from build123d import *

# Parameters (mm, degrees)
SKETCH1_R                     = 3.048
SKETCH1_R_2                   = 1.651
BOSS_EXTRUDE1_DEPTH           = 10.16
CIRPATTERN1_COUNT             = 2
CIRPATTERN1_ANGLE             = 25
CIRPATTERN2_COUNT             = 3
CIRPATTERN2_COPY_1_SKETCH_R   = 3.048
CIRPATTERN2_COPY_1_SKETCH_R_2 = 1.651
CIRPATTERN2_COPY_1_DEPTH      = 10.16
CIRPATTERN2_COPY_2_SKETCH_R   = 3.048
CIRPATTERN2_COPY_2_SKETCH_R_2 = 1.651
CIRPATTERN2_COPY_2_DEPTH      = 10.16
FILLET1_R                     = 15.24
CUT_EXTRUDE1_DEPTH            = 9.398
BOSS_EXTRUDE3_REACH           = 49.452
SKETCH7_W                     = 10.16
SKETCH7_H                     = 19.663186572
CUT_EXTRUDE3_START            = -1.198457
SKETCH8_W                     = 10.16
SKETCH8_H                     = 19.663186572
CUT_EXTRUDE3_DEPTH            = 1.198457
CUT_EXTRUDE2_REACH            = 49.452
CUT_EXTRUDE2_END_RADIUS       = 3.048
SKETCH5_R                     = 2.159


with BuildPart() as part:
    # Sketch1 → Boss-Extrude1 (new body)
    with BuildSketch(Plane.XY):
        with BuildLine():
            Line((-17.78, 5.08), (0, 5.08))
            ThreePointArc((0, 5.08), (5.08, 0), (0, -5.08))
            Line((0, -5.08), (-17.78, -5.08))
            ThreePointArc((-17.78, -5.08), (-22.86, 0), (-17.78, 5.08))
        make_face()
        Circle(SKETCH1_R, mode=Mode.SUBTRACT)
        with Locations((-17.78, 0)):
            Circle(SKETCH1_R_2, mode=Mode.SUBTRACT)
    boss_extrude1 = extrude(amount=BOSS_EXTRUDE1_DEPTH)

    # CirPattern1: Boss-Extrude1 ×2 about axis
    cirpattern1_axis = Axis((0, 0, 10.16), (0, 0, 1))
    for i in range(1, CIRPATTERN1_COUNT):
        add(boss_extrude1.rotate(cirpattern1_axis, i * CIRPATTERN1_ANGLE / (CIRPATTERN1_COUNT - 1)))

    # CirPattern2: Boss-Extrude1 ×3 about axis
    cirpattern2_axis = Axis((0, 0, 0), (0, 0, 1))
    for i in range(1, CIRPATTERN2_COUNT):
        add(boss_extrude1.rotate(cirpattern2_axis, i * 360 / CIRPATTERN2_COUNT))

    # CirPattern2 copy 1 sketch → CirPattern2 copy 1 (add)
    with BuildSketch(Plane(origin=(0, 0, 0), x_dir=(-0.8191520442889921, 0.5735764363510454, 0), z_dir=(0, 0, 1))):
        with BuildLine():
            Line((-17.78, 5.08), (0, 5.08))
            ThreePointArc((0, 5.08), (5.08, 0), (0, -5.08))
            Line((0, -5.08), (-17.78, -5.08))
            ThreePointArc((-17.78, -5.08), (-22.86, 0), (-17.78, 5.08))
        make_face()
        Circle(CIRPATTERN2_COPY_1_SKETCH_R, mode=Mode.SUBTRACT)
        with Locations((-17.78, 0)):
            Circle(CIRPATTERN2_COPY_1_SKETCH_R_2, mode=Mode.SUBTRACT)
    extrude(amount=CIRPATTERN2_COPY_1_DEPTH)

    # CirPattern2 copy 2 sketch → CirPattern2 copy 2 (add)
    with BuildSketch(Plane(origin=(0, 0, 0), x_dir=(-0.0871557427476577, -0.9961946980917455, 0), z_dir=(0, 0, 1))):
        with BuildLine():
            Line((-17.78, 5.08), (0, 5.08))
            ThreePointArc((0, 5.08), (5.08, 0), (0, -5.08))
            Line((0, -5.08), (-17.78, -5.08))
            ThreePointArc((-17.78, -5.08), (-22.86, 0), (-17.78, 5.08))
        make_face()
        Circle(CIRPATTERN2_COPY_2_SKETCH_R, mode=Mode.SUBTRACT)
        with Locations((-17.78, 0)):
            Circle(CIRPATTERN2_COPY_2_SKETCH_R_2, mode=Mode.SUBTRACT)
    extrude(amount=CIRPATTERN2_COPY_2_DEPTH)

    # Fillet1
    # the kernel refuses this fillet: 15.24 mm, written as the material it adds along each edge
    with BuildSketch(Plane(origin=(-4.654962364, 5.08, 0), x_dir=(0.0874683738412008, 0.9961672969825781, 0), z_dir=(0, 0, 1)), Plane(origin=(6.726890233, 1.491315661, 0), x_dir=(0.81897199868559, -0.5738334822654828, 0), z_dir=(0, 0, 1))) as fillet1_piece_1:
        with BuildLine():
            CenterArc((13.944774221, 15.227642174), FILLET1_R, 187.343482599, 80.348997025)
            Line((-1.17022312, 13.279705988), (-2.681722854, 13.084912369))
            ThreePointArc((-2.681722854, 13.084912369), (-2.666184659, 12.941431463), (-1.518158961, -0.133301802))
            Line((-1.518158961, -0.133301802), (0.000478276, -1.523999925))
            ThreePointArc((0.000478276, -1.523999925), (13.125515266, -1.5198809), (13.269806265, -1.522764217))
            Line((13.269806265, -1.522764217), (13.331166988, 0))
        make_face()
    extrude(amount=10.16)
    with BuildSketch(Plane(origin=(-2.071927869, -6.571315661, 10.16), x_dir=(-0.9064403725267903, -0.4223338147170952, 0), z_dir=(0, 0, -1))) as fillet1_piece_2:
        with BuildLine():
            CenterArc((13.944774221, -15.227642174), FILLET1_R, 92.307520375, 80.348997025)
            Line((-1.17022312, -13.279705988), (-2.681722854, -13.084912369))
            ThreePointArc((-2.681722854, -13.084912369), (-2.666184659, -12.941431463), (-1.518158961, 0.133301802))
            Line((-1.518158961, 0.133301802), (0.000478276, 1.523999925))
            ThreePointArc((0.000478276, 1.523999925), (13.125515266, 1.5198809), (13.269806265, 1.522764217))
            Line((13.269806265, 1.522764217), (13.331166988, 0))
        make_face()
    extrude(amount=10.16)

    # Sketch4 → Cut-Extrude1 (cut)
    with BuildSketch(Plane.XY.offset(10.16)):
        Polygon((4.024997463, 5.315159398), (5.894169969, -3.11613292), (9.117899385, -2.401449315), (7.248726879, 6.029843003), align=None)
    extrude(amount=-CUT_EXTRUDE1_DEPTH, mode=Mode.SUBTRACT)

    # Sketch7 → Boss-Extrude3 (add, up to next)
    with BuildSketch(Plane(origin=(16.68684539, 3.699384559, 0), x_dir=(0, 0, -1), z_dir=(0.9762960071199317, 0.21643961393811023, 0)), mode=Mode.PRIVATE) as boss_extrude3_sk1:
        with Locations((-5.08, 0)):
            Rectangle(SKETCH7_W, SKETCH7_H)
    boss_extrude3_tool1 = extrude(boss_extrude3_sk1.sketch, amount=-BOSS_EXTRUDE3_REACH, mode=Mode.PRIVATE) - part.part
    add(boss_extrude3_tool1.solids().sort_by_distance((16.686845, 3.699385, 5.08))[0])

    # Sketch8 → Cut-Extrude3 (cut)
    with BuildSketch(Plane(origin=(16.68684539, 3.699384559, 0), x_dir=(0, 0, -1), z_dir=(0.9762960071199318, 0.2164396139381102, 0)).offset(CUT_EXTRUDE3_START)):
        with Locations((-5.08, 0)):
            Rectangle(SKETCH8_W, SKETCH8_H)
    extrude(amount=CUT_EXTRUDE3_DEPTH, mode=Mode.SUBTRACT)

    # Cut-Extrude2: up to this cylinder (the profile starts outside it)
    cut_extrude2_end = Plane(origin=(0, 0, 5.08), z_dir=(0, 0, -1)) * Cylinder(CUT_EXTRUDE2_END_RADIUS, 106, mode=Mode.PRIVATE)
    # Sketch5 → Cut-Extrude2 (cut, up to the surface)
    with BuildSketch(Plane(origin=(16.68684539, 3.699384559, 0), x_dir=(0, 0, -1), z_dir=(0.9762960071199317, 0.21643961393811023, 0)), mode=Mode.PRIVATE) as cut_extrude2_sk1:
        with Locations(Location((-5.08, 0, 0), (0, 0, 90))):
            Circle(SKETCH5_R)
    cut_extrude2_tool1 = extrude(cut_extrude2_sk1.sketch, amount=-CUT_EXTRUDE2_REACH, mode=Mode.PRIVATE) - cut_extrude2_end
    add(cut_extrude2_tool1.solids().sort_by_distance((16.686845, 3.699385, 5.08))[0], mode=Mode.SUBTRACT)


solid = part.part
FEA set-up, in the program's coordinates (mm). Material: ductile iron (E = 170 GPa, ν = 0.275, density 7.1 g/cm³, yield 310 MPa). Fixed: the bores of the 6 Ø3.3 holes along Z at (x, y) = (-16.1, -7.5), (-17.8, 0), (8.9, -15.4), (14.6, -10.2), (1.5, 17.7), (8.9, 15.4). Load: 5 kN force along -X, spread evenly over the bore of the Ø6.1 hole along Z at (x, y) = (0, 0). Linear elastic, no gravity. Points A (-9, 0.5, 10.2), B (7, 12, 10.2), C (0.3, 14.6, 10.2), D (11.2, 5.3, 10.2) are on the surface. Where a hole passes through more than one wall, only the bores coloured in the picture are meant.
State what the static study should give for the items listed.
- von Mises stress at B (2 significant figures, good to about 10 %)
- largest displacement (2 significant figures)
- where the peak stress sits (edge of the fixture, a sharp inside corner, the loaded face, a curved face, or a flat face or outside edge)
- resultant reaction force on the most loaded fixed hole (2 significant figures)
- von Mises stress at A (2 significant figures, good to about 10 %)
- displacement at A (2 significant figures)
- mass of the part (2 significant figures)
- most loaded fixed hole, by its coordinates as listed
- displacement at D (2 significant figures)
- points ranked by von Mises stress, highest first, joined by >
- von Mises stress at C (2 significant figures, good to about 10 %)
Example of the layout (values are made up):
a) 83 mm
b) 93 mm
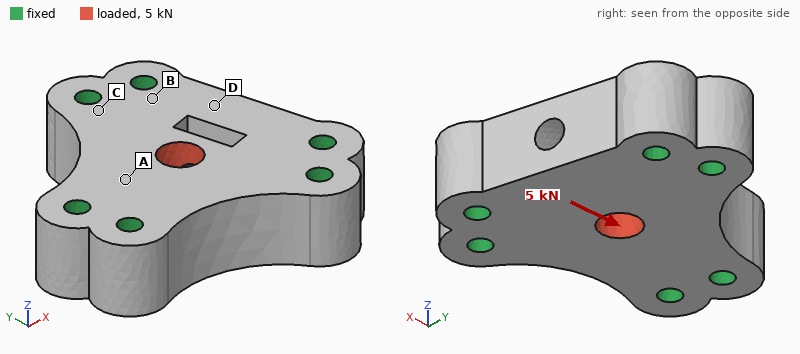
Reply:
a) 17 MPa
b) 4.1 µm
c) the loaded face
d) 1.5 kN
e) 25 MPa
f) 0.96 µm
g) 69 g
h) (-17.8, 0)
i) 0.87 µm
j) A > B > C > D
k) 9.1 MPa
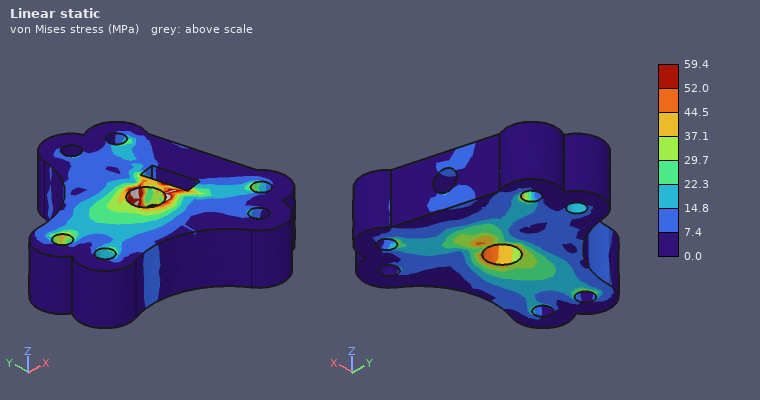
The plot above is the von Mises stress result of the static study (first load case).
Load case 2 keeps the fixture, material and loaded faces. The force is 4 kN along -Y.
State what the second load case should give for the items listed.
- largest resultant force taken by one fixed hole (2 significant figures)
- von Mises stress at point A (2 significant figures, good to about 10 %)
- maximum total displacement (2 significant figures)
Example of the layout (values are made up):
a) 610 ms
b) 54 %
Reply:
a) 1.3 kN
b) 6.4 MPa
c) 2.3 µm
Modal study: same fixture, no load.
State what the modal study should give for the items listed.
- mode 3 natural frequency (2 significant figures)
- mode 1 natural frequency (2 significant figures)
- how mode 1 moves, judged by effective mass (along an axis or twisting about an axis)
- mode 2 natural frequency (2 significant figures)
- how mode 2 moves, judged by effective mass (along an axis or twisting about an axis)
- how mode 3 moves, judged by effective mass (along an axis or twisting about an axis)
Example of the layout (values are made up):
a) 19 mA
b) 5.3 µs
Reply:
a) 54 kHz
b) 40 kHz
c) along Z
d) 51 kHz
e) along Y
f) twisting about Y
